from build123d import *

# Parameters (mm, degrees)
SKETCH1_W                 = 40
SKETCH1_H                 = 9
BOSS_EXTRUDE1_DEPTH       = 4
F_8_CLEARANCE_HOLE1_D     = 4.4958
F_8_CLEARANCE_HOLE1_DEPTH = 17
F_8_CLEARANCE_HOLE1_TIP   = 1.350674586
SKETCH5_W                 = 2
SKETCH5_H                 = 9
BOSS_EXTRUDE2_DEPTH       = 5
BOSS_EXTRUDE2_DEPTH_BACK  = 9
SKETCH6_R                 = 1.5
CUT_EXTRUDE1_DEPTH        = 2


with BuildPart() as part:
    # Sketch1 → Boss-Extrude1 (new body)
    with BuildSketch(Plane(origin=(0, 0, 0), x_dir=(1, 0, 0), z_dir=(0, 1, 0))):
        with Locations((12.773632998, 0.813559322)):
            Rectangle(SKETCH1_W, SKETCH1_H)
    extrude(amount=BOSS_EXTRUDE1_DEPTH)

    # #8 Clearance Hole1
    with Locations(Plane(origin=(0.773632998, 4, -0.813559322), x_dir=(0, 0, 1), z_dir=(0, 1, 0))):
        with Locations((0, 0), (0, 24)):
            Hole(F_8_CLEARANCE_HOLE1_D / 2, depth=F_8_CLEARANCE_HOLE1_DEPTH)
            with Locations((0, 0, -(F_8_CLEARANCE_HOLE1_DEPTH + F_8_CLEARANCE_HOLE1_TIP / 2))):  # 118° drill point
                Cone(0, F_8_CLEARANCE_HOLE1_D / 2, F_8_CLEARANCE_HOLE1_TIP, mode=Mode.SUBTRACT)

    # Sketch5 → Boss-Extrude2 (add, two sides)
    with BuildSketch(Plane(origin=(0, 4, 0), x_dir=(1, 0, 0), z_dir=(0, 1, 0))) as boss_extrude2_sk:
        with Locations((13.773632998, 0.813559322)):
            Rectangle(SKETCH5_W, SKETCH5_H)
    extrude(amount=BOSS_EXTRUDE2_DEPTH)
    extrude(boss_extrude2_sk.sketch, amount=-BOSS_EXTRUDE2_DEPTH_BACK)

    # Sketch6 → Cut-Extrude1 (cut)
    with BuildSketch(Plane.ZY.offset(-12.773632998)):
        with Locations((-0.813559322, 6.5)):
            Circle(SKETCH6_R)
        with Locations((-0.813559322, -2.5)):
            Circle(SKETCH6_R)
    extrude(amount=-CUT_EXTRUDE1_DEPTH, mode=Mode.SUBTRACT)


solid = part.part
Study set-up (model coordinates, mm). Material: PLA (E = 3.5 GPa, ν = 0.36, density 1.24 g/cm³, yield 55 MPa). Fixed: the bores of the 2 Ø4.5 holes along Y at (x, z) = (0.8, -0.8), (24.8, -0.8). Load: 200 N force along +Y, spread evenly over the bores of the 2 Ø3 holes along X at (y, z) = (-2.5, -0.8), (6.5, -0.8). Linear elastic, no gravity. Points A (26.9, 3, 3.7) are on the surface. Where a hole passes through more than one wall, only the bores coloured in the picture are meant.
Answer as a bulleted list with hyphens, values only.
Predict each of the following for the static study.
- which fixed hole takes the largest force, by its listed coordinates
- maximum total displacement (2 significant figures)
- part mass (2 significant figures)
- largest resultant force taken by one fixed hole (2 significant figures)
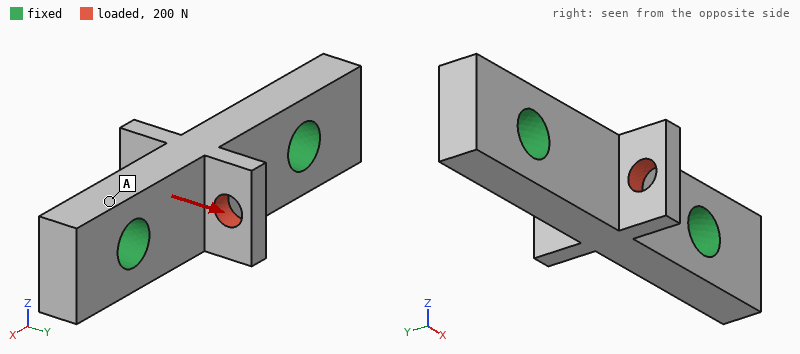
- (24.8, -0.8)
- 95 µm
- 1.8 g
- 110 N
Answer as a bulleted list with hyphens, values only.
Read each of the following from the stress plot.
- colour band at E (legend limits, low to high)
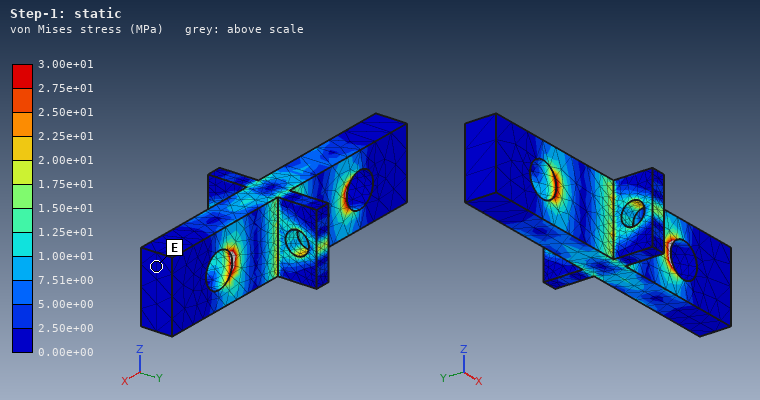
- 0.00e+00 to 2.50e+00 MPa
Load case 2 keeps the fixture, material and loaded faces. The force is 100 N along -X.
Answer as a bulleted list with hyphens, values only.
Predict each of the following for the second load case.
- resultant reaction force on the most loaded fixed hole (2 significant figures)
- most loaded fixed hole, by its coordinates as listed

- 54 N
- (24.8, -0.8)
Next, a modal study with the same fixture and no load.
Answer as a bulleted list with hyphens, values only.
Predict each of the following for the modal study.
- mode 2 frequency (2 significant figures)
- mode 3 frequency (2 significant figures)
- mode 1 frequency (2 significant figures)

- 11 kHz
- 14 kHz
- 11 kHz
